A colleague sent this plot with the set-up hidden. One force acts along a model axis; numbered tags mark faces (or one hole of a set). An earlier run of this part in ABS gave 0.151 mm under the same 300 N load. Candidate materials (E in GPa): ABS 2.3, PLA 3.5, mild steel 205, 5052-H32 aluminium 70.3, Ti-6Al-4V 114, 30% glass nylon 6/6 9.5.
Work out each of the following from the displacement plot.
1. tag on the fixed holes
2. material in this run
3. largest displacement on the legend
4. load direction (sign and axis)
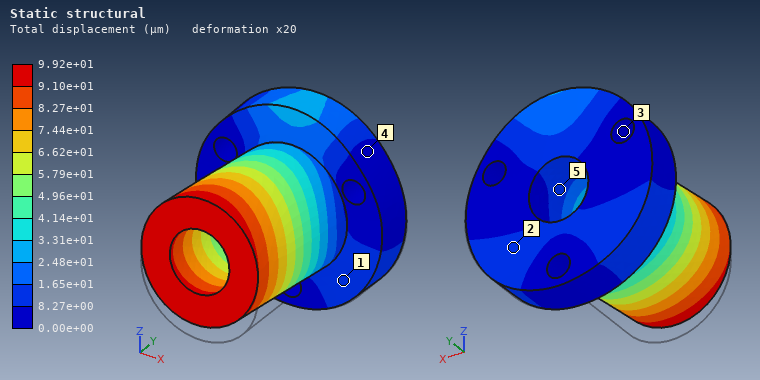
3
PLA
9.92e+01 µm
+Z
